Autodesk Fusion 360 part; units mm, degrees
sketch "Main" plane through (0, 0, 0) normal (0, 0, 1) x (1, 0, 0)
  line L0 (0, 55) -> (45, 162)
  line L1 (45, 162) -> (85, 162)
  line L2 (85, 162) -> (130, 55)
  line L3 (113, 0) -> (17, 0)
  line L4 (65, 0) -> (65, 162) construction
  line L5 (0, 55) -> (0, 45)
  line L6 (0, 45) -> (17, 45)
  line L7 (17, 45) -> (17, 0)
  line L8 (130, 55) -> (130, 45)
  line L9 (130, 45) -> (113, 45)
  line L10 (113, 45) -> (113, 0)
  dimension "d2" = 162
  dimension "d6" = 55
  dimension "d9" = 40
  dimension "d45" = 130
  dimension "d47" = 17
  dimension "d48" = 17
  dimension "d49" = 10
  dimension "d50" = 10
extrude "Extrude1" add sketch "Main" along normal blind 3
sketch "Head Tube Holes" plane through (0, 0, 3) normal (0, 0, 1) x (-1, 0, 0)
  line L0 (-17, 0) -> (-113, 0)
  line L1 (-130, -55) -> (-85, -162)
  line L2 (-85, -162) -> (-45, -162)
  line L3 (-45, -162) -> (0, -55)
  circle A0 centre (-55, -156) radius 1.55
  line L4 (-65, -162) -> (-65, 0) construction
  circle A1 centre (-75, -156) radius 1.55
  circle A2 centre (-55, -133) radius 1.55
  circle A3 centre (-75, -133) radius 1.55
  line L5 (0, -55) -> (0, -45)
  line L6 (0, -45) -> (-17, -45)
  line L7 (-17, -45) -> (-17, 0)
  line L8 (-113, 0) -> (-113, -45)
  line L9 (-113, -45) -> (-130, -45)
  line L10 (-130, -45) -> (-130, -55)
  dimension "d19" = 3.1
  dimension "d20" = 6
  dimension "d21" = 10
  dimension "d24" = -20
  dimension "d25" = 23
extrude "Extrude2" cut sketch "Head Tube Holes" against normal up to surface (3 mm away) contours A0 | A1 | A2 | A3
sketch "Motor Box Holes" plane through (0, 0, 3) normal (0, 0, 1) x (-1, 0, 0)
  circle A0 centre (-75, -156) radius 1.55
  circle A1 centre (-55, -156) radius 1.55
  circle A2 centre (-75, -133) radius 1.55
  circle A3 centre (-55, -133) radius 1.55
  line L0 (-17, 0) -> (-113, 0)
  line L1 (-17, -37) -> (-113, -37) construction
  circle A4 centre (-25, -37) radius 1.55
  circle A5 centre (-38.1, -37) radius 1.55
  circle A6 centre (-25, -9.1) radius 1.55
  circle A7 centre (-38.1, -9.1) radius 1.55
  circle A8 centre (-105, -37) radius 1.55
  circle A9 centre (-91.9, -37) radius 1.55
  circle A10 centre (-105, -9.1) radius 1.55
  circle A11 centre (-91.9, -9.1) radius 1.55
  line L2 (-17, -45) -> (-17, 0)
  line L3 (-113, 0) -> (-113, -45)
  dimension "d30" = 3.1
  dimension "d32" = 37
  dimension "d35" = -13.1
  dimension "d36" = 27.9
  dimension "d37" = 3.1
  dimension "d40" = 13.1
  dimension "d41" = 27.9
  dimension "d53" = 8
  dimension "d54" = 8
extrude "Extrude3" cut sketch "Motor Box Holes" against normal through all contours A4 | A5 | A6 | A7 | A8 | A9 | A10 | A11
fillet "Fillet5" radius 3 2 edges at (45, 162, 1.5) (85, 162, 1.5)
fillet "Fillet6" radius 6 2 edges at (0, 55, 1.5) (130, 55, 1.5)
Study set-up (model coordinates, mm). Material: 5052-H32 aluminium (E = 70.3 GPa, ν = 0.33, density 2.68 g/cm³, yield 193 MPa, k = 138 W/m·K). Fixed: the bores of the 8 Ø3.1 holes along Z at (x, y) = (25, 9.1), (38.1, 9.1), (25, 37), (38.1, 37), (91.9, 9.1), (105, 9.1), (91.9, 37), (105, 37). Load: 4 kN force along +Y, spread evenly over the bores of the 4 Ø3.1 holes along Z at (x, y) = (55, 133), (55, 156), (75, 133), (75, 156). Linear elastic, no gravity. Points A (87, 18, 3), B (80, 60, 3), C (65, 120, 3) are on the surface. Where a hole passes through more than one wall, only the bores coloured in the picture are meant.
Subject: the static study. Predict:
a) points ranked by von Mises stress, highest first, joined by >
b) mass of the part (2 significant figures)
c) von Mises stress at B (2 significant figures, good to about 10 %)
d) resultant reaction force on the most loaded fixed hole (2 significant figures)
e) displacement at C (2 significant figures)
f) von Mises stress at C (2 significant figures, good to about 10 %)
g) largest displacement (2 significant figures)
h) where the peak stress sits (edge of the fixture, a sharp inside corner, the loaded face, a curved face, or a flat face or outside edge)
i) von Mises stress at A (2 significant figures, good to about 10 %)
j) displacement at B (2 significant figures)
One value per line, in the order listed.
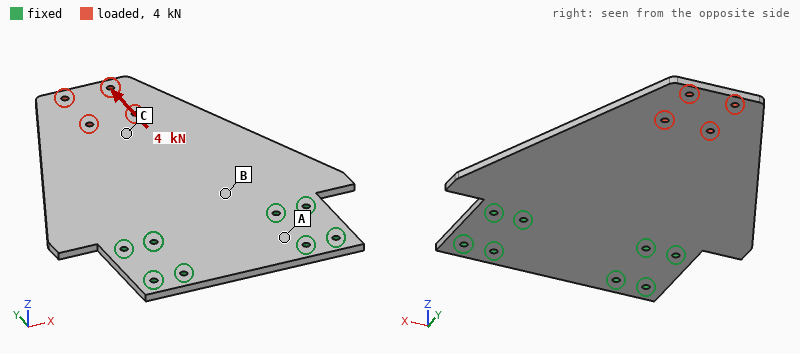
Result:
C > B > A
120 g
14 MPa
860 N
22 µm
22 MPa
32 µm
the loaded face
7.5 MPa
6.5 µm
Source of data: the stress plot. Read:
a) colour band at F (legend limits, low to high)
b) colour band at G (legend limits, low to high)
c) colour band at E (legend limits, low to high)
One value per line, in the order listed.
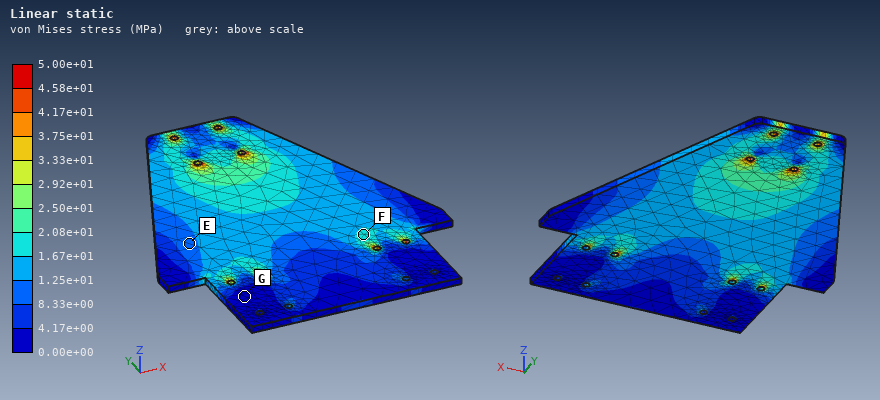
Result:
1.67e+01 to 2.08e+01 MPa
0.00e+00 to 4.17e+00 MPa
8.33e+00 to 1.25e+01 MPa
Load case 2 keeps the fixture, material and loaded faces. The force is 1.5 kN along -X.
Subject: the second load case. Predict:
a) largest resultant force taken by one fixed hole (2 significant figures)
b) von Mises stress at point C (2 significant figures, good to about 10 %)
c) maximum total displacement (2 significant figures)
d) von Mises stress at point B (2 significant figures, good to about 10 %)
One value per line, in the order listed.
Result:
1.4 kN
13 MPa
79 µm
15 MPa
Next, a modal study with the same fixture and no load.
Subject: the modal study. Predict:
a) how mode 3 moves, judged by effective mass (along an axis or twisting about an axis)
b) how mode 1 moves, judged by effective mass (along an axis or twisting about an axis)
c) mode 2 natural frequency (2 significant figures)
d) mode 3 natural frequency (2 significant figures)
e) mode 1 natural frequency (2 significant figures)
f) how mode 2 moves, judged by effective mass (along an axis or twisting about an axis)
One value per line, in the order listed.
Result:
along Z
along Z
740 Hz
1000 Hz
210 Hz
twisting about Y
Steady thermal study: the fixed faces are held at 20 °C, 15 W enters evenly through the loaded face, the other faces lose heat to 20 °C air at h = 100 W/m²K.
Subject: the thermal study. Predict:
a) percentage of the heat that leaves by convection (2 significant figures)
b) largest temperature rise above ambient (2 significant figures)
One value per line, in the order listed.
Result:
86 %
21 K
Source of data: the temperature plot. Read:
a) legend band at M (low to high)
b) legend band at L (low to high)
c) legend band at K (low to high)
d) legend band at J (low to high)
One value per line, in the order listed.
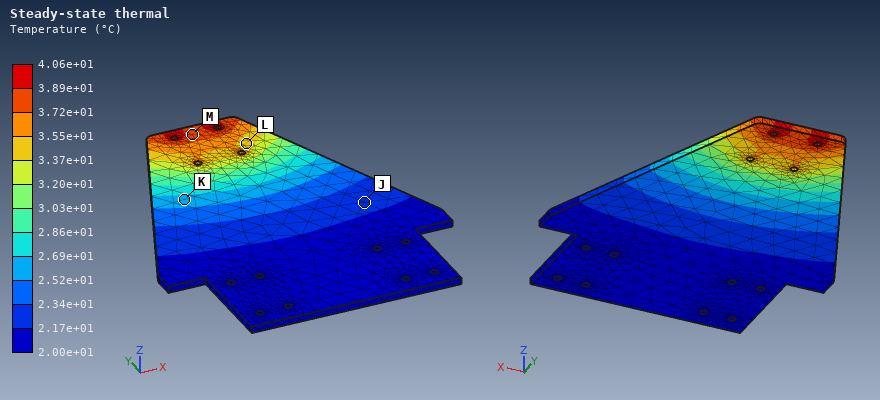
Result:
3.72e+01 to 3.89e+01 °C
3.37e+01 to 3.55e+01 °C
2.52e+01 to 2.69e+01 °C
2.17e+01 to 2.34e+01 °C
